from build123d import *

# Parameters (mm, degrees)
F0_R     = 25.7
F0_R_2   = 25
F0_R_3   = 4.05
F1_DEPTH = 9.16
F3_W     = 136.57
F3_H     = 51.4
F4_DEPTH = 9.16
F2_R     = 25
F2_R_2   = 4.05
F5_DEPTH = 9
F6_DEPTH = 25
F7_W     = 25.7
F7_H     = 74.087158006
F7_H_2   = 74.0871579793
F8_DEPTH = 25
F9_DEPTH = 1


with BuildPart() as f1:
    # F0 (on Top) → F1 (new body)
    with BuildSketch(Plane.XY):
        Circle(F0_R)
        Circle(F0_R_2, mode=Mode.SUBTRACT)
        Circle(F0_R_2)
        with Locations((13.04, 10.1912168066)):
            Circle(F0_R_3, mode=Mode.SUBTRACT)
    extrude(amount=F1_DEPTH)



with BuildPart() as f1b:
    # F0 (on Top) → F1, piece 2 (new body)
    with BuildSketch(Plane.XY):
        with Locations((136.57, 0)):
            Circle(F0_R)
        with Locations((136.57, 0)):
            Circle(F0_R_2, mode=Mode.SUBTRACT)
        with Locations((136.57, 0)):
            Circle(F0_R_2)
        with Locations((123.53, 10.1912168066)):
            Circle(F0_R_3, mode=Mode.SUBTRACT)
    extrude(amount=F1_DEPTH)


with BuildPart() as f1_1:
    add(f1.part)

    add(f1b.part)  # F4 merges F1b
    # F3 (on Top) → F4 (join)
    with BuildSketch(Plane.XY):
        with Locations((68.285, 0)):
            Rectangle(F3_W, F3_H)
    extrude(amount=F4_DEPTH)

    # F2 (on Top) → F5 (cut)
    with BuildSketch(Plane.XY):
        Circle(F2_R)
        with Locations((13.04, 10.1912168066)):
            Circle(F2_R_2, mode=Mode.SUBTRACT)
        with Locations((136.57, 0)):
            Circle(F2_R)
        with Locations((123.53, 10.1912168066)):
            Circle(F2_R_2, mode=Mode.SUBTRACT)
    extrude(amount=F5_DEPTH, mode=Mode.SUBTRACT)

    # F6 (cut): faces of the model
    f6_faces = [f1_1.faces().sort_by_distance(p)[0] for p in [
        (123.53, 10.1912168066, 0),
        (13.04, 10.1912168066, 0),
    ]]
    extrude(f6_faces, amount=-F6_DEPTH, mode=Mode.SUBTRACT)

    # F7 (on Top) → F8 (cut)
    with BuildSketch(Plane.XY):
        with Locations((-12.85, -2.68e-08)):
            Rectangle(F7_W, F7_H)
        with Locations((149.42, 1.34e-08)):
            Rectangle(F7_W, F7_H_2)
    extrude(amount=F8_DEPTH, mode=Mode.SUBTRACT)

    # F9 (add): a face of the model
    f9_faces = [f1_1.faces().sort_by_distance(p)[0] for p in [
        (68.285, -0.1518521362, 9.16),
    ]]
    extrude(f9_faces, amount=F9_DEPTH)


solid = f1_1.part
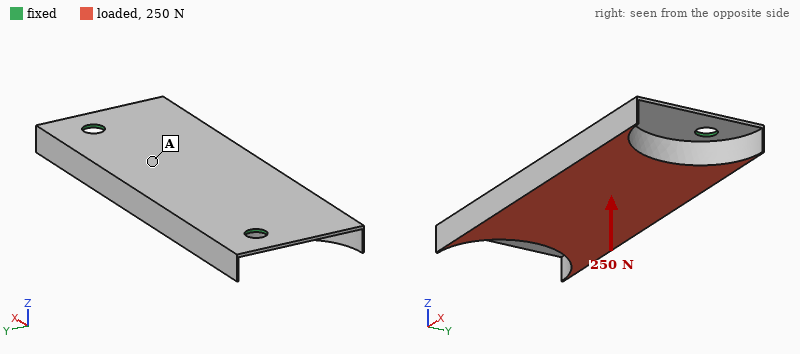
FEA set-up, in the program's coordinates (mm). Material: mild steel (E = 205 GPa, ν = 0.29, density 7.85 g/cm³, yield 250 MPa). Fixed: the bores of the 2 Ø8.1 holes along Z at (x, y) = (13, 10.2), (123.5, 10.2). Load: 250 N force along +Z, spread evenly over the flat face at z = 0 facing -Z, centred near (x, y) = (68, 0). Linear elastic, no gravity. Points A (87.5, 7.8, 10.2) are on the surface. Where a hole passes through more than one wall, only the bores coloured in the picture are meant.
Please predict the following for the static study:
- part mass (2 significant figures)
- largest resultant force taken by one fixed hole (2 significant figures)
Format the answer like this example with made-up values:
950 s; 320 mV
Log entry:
420 g; 200 N
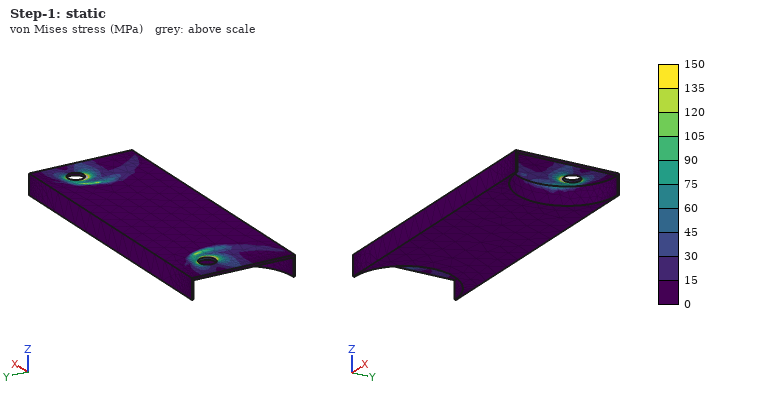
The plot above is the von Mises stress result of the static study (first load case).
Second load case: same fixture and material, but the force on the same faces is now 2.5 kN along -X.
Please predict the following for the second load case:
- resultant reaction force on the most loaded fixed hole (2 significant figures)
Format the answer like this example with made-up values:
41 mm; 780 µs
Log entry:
1.3 kN
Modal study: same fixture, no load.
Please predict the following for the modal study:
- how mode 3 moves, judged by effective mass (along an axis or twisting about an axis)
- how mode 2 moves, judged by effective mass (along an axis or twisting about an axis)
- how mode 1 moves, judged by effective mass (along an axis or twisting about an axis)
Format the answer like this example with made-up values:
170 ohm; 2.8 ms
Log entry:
twisting about Y; along Z; along Z
